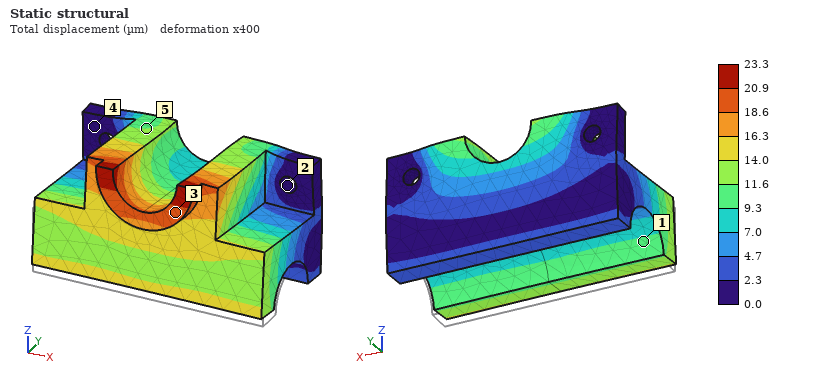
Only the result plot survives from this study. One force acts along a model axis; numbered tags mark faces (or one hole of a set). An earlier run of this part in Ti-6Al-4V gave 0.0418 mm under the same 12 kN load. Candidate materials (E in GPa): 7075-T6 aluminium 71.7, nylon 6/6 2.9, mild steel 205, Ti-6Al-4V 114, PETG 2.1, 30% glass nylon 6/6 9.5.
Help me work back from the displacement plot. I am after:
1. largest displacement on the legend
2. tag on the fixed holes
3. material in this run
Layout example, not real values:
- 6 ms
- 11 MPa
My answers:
- 23.3 µm
- 2
- mild steel
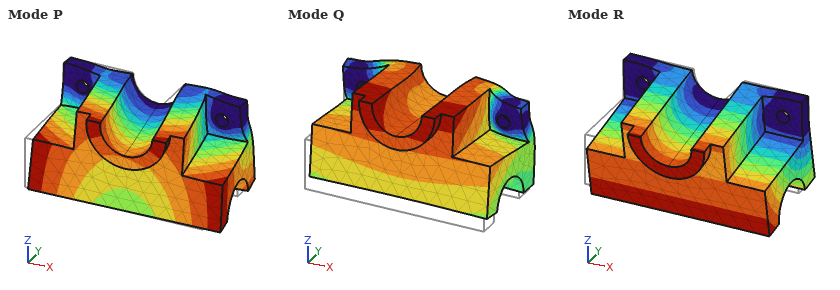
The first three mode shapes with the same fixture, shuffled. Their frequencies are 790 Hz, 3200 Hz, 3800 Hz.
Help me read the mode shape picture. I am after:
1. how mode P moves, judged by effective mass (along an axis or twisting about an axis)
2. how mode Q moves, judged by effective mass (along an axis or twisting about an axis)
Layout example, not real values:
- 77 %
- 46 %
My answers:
- along X
- along Y
